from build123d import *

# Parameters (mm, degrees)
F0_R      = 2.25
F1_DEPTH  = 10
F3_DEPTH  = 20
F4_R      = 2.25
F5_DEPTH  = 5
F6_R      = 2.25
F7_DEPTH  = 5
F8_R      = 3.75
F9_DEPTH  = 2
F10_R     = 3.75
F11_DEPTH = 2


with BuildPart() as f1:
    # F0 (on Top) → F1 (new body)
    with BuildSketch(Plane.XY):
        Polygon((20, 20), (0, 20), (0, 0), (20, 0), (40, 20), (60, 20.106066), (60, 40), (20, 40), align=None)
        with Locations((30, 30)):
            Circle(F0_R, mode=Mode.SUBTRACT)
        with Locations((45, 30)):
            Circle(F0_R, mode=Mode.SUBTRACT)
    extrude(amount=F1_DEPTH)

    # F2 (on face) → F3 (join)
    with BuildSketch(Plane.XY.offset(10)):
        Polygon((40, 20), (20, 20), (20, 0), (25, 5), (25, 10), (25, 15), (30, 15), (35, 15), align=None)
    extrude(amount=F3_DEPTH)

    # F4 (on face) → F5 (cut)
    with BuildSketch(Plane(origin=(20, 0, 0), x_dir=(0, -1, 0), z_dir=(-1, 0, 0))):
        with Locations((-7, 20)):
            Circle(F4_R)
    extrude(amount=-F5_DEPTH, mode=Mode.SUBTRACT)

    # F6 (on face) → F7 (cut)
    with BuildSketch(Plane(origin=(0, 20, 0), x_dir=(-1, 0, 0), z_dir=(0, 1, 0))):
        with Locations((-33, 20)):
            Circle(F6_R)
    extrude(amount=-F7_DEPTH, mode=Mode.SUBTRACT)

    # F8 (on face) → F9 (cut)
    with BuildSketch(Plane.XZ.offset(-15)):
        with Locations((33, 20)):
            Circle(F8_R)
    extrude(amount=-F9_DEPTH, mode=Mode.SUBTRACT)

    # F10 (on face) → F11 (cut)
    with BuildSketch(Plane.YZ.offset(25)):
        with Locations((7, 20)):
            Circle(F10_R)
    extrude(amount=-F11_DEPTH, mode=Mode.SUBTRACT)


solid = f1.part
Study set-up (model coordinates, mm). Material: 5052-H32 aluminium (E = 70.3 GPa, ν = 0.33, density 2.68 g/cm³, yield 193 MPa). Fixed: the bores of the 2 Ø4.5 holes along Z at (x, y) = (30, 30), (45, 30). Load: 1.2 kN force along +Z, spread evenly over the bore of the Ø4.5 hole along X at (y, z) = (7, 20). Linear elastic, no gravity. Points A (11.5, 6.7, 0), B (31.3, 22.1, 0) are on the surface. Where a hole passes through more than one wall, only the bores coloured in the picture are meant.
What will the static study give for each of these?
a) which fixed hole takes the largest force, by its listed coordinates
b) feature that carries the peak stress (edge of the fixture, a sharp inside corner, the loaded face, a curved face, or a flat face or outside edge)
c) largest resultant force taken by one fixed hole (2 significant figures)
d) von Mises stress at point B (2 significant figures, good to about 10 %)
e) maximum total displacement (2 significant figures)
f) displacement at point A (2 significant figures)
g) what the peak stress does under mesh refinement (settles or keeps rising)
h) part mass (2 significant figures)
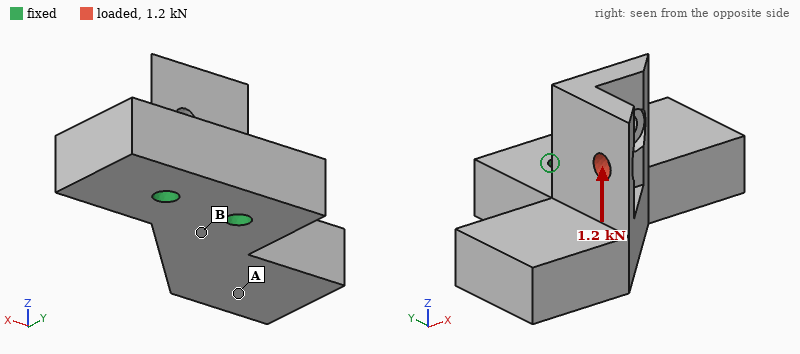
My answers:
(30, 30)
edge of the fixture
1.4 kN
59 MPa
0.12 mm
0.068 mm
keeps rising
44 g
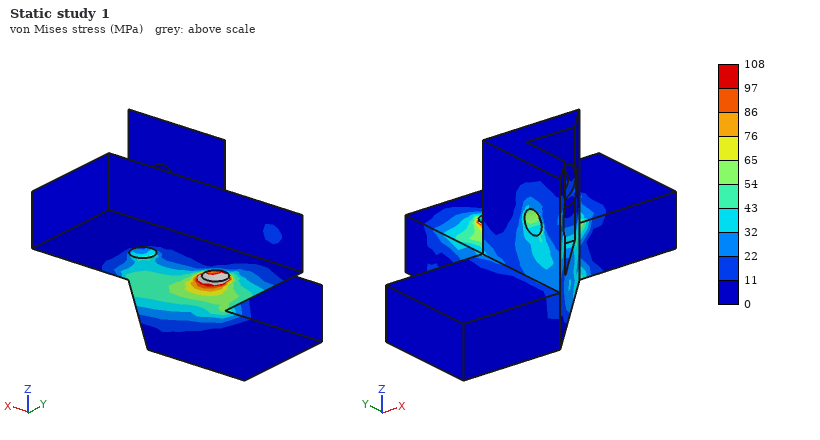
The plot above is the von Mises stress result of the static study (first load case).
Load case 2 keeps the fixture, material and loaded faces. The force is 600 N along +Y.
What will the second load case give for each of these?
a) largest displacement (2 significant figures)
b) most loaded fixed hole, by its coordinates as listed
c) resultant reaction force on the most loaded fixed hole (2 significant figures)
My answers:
57 µm
(30, 30)
840 N
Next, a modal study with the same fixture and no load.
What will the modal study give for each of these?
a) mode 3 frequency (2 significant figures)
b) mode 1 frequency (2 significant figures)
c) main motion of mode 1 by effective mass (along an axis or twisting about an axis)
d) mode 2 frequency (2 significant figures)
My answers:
8100 Hz
4500 Hz
along Z
6900 Hz
